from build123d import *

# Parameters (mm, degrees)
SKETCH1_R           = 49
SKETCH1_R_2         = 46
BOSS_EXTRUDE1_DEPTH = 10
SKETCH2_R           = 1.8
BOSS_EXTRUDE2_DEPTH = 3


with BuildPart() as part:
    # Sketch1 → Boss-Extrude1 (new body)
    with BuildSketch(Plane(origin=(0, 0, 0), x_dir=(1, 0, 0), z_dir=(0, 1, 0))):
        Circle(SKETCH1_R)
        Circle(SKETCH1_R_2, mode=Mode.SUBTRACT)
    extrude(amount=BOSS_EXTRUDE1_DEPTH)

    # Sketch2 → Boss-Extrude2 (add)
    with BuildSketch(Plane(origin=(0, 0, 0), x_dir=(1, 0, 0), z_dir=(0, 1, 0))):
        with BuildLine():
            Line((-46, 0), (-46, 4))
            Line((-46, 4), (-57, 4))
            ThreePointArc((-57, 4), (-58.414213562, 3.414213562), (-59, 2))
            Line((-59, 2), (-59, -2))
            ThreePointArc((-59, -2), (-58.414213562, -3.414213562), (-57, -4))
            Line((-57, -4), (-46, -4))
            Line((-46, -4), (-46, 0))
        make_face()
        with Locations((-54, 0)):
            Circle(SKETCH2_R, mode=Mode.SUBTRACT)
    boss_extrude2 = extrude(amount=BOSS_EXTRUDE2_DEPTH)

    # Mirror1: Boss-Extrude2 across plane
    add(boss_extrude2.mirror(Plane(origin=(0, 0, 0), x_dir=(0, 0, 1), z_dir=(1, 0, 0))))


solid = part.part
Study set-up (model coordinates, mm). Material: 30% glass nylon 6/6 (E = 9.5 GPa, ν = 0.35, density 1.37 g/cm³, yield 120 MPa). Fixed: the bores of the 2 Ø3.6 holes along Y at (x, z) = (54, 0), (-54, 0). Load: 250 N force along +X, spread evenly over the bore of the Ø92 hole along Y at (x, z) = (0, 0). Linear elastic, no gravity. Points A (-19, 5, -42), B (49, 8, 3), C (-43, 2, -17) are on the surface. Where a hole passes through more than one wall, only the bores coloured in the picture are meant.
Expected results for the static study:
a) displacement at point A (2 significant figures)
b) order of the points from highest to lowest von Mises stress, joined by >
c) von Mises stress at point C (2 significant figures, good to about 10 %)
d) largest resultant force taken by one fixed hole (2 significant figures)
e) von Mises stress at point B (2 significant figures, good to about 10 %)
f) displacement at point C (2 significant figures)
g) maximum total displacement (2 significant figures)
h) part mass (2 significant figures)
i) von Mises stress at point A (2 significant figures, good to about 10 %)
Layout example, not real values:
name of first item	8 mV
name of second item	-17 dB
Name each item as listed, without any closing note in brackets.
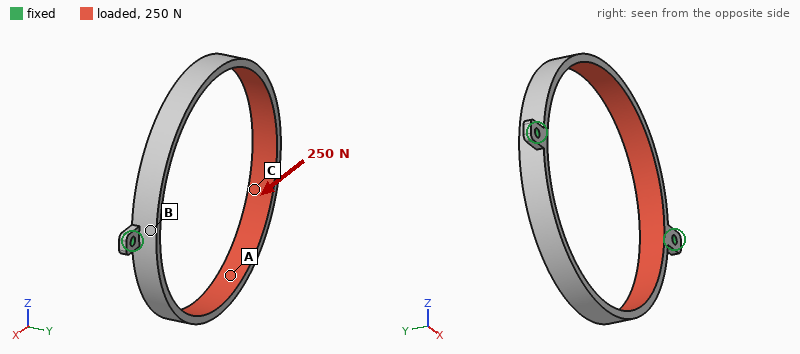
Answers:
displacement at point A	1.0 mm
order of the points from highest to lowest von Mises stress, joined by >	B > A > C
von Mises stress at point C	6.9 MPa
largest resultant force taken by one fixed hole	130 N
von Mises stress at point B	38 MPa
displacement at point C	0.40 mm
maximum total displacement	1.1 mm
part mass	13 g
von Mises stress at point A	24 MPa
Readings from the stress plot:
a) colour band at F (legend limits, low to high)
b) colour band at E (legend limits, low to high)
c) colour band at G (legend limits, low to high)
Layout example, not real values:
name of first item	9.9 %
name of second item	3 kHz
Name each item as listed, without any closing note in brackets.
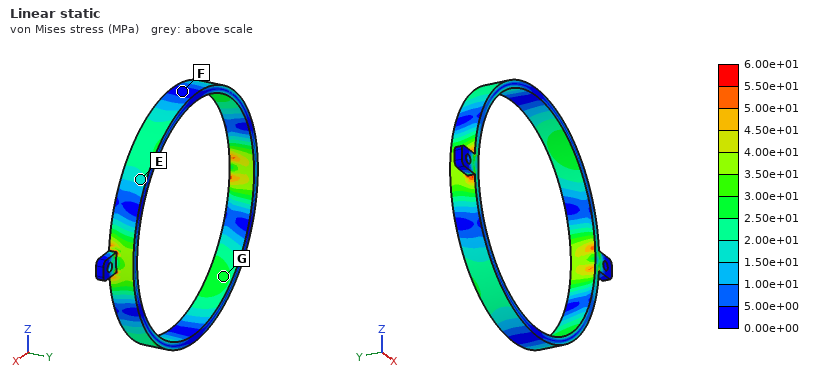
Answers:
colour band at F	0.00e+00 to 5.00e+00 MPa
colour band at E	1.50e+01 to 2.00e+01 MPa
colour band at G	2.50e+01 to 3.00e+01 MPa
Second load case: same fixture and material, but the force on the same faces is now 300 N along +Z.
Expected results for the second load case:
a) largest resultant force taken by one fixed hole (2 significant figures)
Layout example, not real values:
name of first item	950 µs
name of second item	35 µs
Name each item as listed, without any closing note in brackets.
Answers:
largest resultant force taken by one fixed hole	150 N
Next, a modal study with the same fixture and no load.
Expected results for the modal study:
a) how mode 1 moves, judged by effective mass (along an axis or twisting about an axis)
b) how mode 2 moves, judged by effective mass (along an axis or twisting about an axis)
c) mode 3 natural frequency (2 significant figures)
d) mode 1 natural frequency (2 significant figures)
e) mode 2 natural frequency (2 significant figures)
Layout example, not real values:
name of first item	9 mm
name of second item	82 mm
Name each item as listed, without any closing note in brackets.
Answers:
how mode 1 moves, judged by effective mass	twisting about X
how mode 2 moves, judged by effective mass	along Y
mode 3 natural frequency	670 Hz
mode 1 natural frequency	370 Hz
mode 2 natural frequency	630 Hz
